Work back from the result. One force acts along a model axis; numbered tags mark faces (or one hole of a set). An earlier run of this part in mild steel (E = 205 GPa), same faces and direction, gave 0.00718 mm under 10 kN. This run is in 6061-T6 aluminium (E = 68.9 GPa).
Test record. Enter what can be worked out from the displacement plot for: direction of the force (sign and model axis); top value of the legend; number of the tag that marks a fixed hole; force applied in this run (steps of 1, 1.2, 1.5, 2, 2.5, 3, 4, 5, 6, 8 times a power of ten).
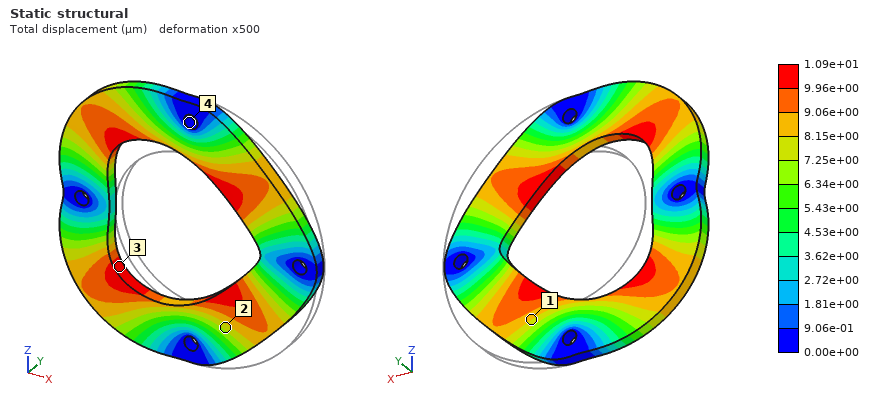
-X
1.09e+01 µm
4
5 kN
